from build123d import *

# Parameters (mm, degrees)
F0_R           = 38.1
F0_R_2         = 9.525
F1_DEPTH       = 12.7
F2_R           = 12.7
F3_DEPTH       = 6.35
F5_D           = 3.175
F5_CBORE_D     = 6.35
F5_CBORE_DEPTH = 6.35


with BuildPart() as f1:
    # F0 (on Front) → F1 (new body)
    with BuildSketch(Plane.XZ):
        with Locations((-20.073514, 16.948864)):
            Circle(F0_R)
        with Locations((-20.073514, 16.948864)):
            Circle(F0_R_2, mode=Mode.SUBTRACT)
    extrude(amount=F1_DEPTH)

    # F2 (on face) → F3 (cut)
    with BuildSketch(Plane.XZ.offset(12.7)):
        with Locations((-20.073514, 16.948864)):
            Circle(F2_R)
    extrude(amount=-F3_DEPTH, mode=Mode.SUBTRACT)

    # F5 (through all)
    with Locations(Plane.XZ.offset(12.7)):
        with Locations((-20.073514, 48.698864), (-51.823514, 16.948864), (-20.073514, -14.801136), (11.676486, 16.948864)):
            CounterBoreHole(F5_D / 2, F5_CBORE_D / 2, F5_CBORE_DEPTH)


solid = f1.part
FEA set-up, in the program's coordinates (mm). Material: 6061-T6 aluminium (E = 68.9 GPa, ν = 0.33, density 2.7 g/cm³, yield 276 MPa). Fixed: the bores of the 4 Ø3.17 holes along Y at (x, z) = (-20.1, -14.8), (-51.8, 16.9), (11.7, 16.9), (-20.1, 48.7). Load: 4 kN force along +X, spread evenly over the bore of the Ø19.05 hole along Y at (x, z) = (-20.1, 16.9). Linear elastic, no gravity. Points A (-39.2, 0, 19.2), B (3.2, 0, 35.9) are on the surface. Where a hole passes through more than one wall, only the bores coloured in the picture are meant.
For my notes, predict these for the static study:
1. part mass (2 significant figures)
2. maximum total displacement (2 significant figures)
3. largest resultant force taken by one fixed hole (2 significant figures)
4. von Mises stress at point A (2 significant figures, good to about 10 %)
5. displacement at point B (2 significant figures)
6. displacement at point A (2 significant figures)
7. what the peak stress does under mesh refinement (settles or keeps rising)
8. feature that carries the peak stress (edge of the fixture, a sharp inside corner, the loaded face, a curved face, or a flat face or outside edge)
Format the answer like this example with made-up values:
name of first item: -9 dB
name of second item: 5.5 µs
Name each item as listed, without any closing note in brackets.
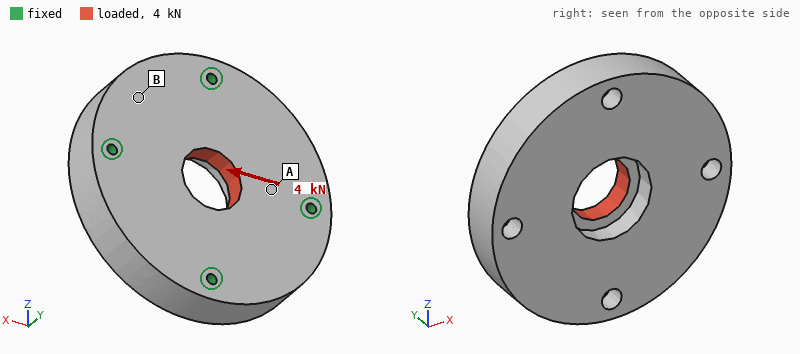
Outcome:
part mass: 140 g
maximum total displacement: 4.0 µm
largest resultant force taken by one fixed hole: 1.2 kN
von Mises stress at point A: 11 MPa
displacement at point B: 1.9 µm
displacement at point A: 2.3 µm
what the peak stress does under mesh refinement: keeps rising
feature that carries the peak stress: edge of the fixture
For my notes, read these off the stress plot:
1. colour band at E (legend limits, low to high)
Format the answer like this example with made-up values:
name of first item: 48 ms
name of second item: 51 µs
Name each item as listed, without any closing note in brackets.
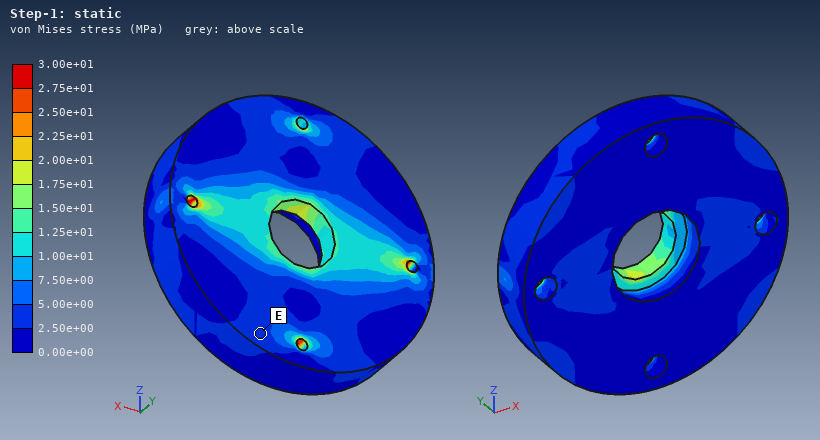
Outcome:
colour band at E: 2.50e+00 to 5.00e+00 MPa
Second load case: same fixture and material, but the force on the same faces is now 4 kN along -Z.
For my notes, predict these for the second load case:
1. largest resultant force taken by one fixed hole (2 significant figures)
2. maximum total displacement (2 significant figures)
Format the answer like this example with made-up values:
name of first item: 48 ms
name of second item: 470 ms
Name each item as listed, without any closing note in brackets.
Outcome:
largest resultant force taken by one fixed hole: 1.2 kN
maximum total displacement: 4.0 µm
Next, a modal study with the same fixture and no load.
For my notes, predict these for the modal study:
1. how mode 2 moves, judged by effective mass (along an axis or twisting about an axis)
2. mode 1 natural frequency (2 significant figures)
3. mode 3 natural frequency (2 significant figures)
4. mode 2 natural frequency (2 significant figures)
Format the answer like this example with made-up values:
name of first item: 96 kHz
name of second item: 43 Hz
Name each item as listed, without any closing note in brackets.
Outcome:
how mode 2 moves, judged by effective mass: along Y
mode 1 natural frequency: 12 kHz
mode 3 natural frequency: 14 kHz
mode 2 natural frequency: 13 kHz
